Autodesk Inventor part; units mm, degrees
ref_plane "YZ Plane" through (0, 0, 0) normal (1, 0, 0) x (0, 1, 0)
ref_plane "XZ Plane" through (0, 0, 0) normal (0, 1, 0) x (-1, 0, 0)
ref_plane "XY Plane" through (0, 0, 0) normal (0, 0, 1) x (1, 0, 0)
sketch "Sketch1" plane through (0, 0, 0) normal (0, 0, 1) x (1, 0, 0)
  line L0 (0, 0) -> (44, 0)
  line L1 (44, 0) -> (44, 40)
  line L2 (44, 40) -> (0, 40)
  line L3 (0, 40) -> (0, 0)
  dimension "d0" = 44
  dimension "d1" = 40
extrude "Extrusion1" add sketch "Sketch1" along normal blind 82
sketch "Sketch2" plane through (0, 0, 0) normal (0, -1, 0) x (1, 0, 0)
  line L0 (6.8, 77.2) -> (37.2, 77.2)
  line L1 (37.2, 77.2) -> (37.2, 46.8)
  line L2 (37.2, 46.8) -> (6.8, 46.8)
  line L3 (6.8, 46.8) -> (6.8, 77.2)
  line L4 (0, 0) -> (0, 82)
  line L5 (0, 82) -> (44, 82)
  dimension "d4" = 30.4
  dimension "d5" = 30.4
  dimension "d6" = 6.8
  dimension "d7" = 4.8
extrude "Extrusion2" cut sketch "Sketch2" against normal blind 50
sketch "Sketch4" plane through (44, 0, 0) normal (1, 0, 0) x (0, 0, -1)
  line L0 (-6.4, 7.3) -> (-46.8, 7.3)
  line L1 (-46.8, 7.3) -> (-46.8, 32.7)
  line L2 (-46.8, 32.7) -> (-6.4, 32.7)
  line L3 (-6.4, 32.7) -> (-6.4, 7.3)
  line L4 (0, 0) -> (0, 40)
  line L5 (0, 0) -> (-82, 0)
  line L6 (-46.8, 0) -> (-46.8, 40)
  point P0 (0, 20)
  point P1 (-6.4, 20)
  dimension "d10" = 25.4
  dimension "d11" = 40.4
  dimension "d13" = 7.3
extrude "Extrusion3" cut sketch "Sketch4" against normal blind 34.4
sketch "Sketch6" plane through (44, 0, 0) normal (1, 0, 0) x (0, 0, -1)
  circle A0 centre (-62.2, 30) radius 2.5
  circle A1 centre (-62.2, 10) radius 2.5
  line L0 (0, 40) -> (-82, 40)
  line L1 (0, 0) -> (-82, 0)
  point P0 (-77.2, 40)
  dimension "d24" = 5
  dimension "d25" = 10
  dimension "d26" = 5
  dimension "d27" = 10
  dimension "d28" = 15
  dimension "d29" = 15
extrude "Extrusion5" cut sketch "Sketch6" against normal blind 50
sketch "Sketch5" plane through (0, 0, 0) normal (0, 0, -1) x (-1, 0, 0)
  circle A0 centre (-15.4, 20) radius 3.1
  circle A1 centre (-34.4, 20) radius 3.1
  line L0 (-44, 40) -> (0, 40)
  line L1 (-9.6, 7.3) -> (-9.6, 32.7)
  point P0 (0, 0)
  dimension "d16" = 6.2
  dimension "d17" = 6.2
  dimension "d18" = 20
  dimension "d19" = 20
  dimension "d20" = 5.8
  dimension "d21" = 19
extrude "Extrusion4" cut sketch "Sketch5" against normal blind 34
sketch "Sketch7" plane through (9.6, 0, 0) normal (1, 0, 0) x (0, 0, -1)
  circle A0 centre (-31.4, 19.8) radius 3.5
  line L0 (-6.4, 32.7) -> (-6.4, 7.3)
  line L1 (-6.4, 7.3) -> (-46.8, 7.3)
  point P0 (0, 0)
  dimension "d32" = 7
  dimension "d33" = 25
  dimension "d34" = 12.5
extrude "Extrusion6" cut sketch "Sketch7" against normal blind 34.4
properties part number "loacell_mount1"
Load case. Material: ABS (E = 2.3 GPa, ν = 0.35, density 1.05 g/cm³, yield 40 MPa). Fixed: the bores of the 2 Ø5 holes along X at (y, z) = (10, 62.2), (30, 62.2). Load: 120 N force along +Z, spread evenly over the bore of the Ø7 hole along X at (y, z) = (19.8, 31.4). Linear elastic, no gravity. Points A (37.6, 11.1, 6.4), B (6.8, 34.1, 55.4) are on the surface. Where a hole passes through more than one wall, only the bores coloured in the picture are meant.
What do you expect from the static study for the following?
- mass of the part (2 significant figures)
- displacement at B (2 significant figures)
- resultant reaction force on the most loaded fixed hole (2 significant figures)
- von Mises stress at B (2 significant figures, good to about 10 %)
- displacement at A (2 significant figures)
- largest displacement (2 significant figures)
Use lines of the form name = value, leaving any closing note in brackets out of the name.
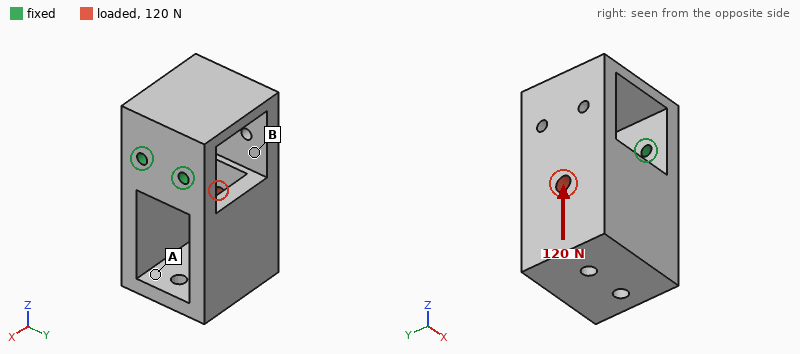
mass of the part = 74 g
displacement at B = 0.58 mm
resultant reaction force on the most loaded fixed hole = 62 N
von Mises stress at B = 2.3 MPa
displacement at A = 0.78 mm
largest displacement = 1.1 mm
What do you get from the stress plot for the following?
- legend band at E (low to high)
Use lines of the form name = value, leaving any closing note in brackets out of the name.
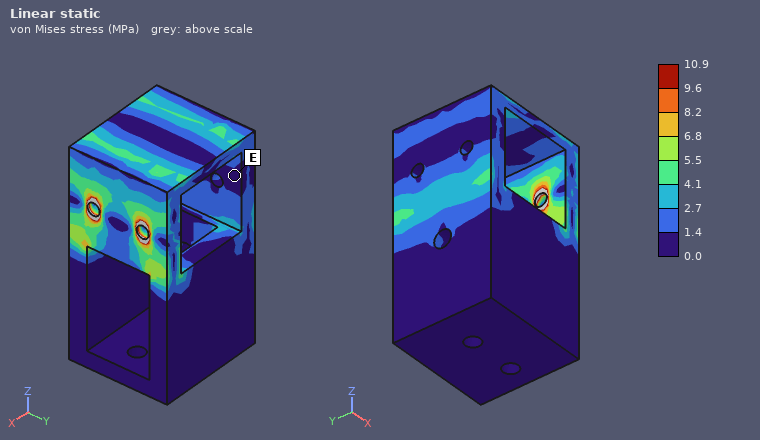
legend band at E = 0.0 to 1.4 MPa
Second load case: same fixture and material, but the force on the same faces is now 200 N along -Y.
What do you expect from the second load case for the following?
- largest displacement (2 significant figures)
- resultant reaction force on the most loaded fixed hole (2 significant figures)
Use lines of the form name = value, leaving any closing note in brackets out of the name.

largest displacement = 0.74 mm
resultant reaction force on the most loaded fixed hole = 380 N
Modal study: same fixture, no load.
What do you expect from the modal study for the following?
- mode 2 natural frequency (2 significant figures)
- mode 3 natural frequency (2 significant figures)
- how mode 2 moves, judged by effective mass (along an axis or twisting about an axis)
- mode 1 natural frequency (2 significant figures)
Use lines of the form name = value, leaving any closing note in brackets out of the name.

mode 2 natural frequency = 420 Hz
mode 3 natural frequency = 770 Hz
how mode 2 moves, judged by effective mass = along Y
mode 1 natural frequency = 240 Hz
